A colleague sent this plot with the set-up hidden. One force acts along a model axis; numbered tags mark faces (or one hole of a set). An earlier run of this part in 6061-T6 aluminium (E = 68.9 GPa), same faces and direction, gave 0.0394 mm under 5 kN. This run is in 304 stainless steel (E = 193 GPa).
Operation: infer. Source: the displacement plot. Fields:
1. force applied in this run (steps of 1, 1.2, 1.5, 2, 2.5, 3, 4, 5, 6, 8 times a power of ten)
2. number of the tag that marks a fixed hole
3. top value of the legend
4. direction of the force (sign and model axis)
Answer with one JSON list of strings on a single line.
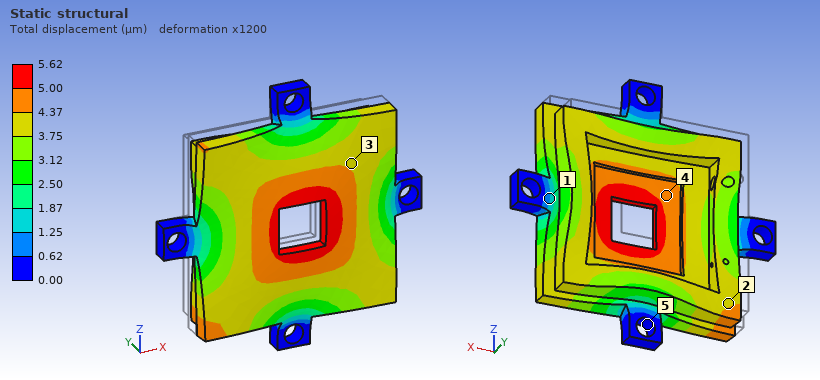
["2 kN", "5", "5.62 µm", "-Y"]
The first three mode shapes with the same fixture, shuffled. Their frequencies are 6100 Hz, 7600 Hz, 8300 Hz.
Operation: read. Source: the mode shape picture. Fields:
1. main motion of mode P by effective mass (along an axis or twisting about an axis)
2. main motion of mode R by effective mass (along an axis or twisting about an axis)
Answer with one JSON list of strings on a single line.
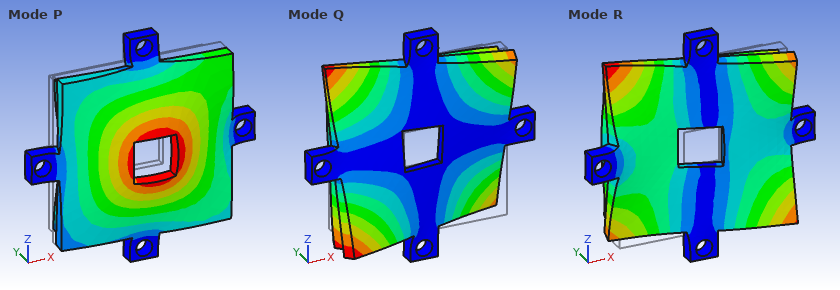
["along Y", "twisting about Z"]
